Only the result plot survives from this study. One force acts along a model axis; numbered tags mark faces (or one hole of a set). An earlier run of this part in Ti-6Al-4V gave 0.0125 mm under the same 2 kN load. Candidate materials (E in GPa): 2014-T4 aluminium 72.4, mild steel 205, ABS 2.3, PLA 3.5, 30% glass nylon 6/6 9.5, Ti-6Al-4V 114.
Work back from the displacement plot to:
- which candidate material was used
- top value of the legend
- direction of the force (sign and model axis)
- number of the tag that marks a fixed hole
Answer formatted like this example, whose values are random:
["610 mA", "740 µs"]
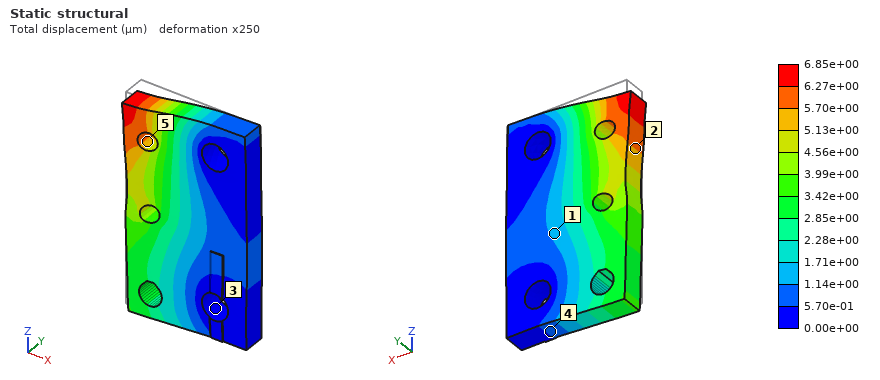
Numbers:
["mild steel", "6.85e+00 µm", "-Z", "3"]
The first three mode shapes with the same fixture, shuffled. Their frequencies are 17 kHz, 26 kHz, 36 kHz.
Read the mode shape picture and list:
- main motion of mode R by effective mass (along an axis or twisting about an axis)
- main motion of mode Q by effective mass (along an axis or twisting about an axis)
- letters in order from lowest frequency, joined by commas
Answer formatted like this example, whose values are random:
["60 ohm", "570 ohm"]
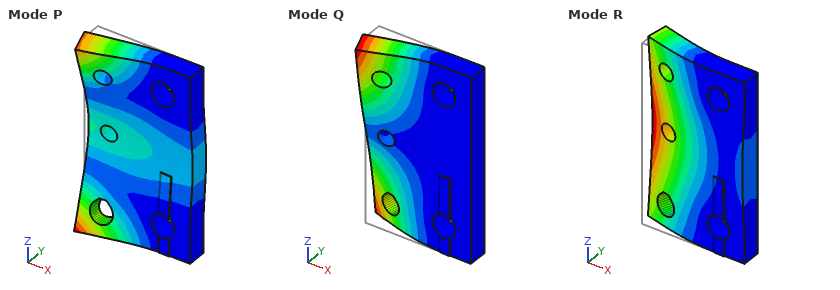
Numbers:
["along Y", "twisting about X", "R, Q, P"]
